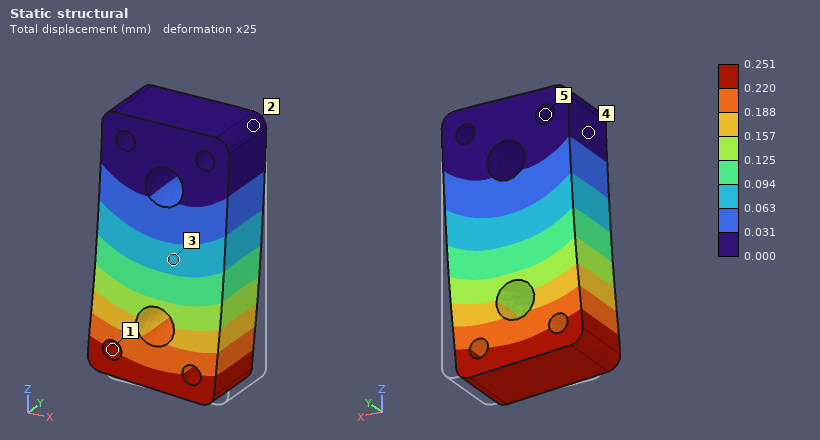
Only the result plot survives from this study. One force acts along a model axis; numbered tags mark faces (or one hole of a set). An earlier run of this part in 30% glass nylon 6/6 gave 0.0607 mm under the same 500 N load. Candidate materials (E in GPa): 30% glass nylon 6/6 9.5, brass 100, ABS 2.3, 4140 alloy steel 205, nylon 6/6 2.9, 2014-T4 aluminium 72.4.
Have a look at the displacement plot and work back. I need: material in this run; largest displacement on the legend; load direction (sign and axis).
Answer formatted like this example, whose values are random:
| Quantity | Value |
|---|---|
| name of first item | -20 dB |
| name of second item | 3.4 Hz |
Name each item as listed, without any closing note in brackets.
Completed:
| Quantity | Value |
|---|---|
| material in this run | ABS |
| largest displacement on the legend | 0.251 mm |
| load direction | -X |
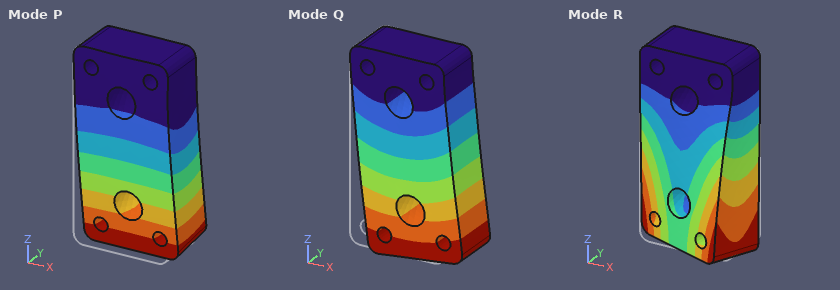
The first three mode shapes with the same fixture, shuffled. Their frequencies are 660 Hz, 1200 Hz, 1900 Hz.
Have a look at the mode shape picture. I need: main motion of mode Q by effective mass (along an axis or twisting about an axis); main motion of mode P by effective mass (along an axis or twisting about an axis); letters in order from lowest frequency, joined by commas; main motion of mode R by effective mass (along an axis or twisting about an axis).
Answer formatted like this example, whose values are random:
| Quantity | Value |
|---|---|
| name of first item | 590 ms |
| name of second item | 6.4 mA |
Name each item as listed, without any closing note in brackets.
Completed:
| Quantity | Value |
|---|---|
| main motion of mode Q by effective mass | along X |
| main motion of mode P by effective mass | along Y |
| letters in order from lowest frequency, joined by commas | P, Q, R |
| main motion of mode R by effective mass | twisting about Z |
